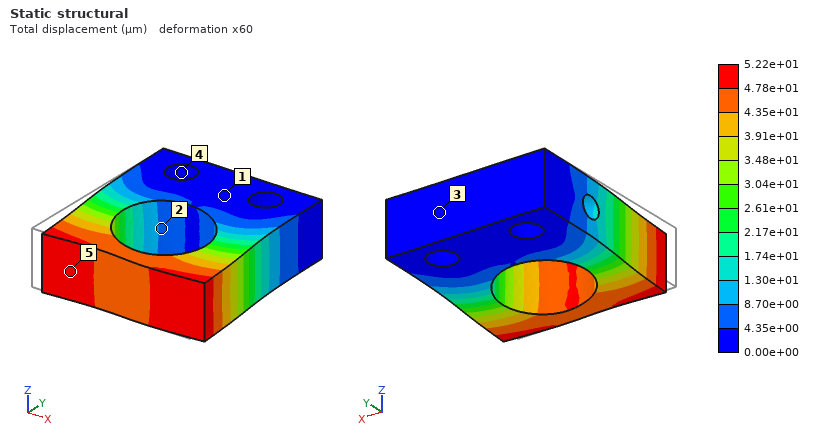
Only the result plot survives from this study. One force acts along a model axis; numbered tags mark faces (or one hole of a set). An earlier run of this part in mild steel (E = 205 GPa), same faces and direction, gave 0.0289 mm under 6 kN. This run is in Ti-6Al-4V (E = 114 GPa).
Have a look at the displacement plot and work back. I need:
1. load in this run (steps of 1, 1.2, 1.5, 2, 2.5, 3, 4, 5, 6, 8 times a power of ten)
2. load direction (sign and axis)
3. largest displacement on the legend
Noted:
6 kN
+X
5.22e+01 µm
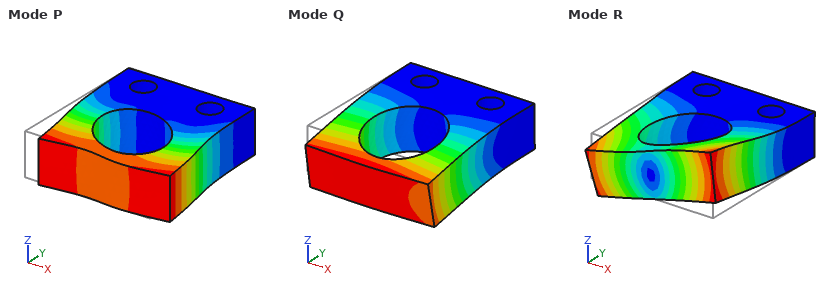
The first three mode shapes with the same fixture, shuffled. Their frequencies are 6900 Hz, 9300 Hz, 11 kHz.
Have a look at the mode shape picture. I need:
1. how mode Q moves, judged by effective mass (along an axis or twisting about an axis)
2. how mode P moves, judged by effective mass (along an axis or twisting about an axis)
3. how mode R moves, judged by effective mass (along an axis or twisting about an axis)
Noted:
along Z
along X
twisting about Y
